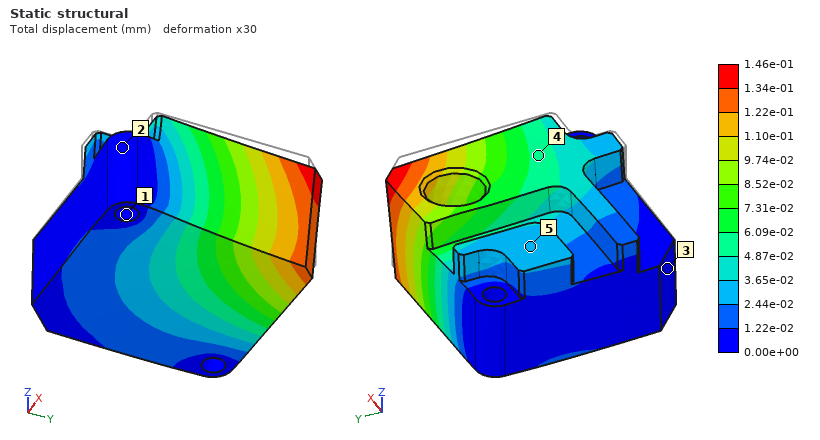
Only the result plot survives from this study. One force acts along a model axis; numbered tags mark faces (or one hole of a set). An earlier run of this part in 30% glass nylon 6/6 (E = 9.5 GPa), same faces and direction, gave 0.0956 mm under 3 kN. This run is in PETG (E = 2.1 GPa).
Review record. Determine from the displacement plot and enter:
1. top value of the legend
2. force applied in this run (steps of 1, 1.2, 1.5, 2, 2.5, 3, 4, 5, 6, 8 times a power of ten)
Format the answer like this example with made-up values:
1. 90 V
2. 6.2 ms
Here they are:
1. 1.46e-01 mm
2. 1 kN
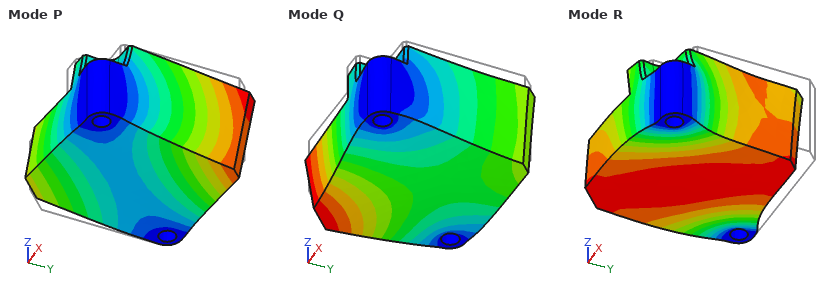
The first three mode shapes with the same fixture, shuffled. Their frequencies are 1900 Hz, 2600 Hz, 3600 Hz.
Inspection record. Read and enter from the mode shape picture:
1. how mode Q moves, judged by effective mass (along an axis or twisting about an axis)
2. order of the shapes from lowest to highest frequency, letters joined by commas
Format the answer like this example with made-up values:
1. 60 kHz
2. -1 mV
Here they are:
1. along Z
2. P, Q, R
